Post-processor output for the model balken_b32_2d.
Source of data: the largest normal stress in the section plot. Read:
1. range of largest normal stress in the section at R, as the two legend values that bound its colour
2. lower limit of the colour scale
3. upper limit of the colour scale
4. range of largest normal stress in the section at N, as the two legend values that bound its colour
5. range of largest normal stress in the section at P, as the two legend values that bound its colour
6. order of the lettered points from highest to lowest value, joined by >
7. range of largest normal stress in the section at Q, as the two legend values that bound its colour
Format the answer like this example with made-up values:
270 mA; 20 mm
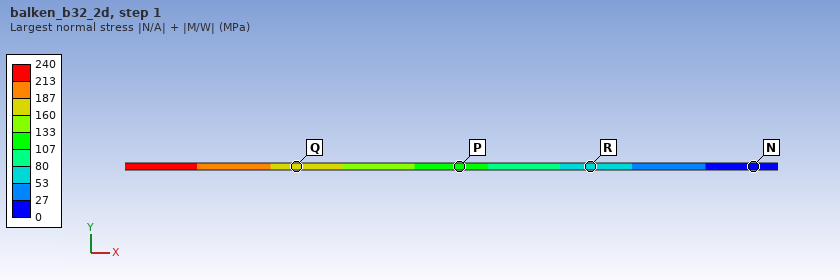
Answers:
53 to 80 MPa; 0 MPa; 240 MPa; 0 to 27 MPa; 107 to 133 MPa; Q > P > R > N; 160 to 187 MPa
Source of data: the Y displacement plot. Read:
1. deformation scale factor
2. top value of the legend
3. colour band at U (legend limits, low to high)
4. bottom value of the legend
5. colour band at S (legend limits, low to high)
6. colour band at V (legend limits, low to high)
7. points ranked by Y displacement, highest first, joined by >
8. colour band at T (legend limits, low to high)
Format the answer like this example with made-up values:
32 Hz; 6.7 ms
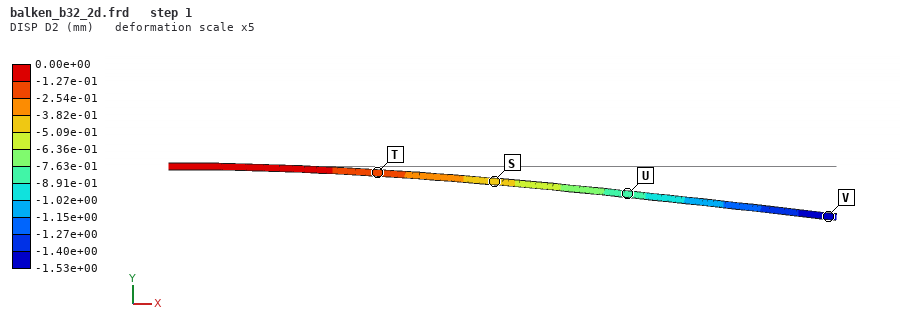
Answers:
5; 0.00e+00 mm; -8.91e-01 to -7.63e-01 mm; -1.53e+00 mm; -5.09e-01 to -3.82e-01 mm; -1.53e+00 to -1.40e+00 mm; T > S > U > V; -2.54e-01 to -1.27e-01 mm
